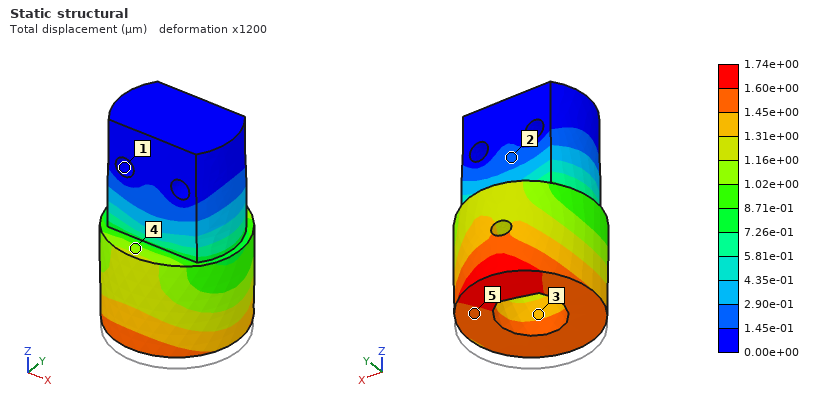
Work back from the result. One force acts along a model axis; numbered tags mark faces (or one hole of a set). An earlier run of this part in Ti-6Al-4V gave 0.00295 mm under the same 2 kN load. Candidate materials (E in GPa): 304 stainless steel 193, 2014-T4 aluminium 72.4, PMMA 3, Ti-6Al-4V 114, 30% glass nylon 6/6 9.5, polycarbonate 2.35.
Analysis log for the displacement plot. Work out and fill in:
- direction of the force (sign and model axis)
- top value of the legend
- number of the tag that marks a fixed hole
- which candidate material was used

+Z
1.74e+00 µm
1
304 stainless steel
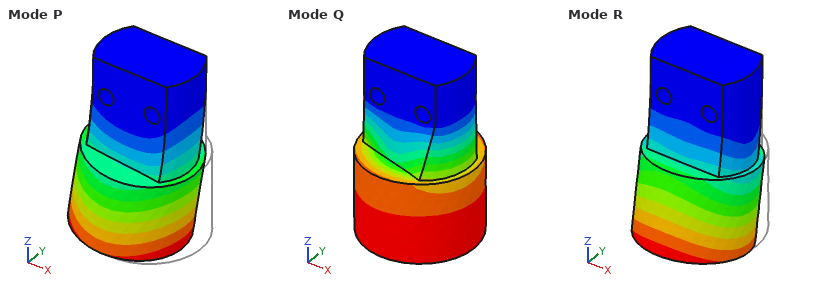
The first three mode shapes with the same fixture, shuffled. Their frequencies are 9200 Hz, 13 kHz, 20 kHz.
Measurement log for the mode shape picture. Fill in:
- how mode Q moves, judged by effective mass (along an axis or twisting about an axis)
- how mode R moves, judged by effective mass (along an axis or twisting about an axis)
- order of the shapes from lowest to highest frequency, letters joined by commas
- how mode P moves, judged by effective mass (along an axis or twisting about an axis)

twisting about Z
along Y
R, P, Q
along X
